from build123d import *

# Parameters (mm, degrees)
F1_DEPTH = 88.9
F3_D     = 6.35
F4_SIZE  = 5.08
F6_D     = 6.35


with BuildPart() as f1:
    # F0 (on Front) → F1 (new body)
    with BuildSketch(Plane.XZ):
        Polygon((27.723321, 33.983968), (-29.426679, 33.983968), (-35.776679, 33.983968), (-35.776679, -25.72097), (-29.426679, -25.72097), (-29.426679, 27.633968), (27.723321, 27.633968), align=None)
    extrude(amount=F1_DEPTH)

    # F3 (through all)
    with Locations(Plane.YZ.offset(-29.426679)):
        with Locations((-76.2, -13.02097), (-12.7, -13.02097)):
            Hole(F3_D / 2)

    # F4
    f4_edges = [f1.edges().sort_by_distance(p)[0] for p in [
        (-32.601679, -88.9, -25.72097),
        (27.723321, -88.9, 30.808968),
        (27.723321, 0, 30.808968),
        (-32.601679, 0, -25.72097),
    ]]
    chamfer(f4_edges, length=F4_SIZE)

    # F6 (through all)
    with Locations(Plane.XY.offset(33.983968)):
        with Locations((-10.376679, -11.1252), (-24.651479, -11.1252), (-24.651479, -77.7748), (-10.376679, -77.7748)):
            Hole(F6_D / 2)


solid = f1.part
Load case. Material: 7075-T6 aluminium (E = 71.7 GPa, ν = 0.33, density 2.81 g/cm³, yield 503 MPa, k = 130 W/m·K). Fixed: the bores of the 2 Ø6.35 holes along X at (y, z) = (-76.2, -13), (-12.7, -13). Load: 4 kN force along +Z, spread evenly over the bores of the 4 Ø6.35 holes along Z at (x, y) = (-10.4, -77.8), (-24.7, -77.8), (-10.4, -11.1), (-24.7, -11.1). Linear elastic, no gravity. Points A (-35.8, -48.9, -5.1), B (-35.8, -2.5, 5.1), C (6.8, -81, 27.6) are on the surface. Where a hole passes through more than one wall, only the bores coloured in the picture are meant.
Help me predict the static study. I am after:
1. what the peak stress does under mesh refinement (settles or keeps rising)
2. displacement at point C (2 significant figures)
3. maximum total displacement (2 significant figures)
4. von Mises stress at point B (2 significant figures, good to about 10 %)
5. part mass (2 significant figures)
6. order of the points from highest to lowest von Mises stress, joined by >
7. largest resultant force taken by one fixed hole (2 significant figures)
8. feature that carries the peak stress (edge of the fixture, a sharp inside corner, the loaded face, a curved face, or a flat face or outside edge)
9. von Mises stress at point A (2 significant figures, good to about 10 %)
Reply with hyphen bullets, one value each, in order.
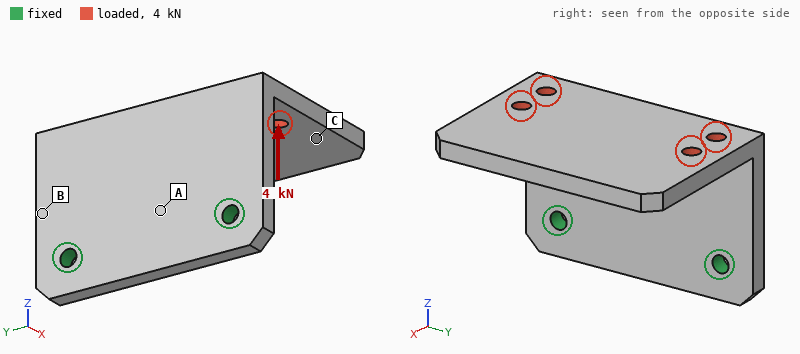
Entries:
- keeps rising
- 0.99 mm
- 1.5 mm
- 110 MPa
- 180 g
- B > A > C
- 2.0 kN
- edge of the fixture
- 58 MPa
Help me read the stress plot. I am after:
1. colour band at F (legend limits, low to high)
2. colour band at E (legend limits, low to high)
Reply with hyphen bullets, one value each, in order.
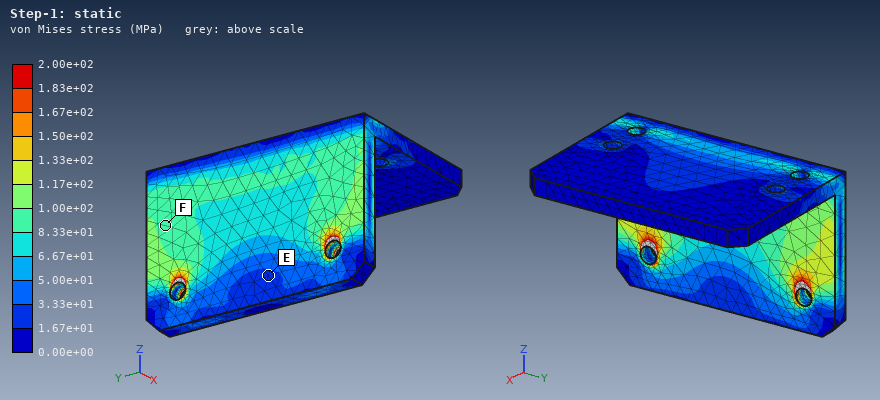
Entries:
- 8.33e+01 to 1.00e+02 MPa
- 1.67e+01 to 3.33e+01 MPa
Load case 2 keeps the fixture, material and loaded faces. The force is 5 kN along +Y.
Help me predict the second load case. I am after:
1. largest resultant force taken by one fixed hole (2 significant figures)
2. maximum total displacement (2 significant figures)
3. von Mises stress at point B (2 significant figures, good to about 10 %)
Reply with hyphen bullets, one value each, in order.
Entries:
- 4.3 kN
- 0.51 mm
- 64 MPa
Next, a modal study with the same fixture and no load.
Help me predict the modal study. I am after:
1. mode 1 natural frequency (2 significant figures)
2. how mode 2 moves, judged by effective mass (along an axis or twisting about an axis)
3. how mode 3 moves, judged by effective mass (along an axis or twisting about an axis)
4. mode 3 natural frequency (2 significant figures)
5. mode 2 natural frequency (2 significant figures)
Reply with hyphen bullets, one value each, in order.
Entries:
- 610 Hz
- along Y
- along X
- 1700 Hz
- 1200 Hz
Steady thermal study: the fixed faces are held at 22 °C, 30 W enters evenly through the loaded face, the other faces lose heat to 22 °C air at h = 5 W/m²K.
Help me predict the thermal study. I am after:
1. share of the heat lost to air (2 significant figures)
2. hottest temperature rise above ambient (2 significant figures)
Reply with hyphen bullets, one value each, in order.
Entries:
- 6.4 %
- 28 K
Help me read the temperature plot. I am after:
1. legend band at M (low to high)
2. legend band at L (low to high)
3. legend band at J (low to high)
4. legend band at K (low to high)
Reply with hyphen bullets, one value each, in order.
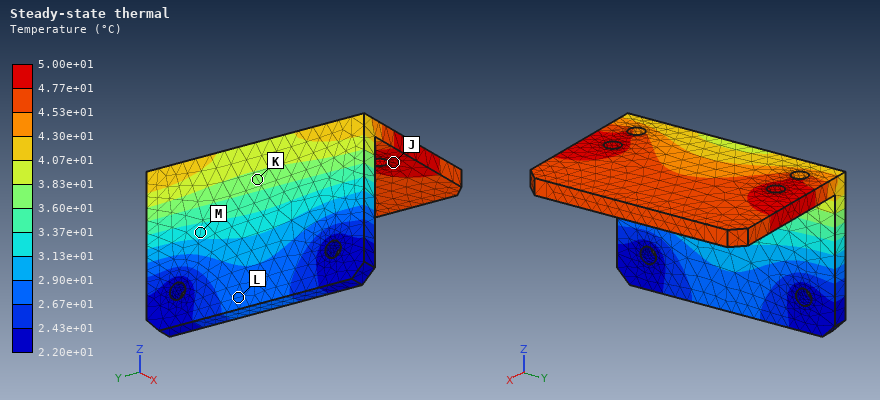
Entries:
- 3.13e+01 to 3.37e+01 °C
- 2.67e+01 to 2.90e+01 °C
- 4.77e+01 to 5.00e+01 °C
- 3.60e+01 to 3.83e+01 °C
